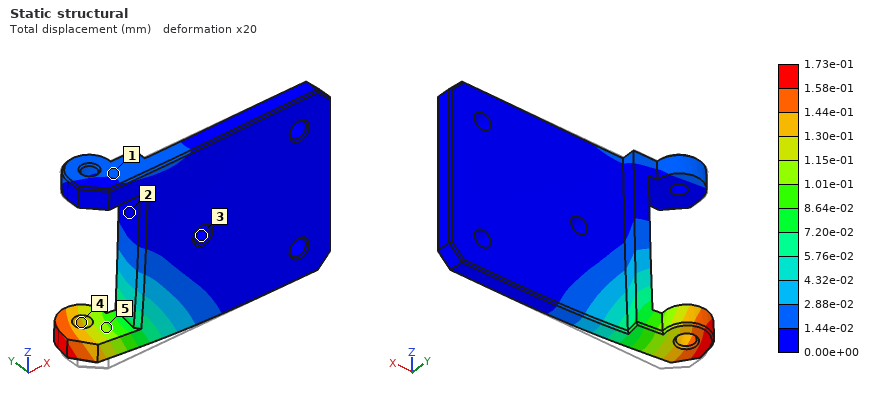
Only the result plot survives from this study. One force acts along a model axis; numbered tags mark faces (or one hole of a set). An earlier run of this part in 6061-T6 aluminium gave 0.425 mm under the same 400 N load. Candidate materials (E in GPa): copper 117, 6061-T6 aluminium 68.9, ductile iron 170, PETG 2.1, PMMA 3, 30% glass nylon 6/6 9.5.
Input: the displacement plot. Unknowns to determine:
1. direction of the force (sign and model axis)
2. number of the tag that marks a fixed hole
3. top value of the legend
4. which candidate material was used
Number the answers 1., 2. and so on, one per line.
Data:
1. +Y
2. 3
3. 1.73e-01 mm
4. ductile iron
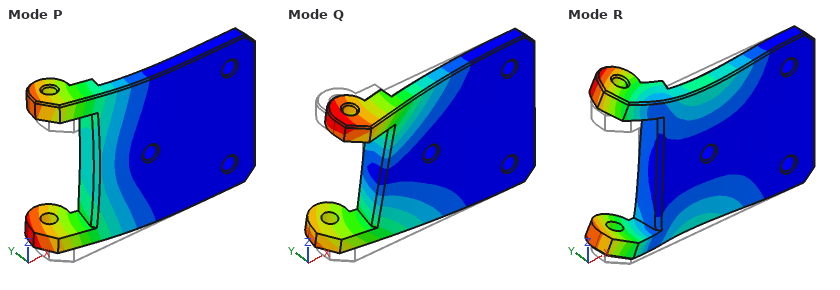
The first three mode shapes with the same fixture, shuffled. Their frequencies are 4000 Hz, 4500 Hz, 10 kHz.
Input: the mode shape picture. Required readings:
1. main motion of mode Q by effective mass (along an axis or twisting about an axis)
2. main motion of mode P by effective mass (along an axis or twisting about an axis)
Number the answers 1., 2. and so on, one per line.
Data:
1. twisting about X
2. along Y
